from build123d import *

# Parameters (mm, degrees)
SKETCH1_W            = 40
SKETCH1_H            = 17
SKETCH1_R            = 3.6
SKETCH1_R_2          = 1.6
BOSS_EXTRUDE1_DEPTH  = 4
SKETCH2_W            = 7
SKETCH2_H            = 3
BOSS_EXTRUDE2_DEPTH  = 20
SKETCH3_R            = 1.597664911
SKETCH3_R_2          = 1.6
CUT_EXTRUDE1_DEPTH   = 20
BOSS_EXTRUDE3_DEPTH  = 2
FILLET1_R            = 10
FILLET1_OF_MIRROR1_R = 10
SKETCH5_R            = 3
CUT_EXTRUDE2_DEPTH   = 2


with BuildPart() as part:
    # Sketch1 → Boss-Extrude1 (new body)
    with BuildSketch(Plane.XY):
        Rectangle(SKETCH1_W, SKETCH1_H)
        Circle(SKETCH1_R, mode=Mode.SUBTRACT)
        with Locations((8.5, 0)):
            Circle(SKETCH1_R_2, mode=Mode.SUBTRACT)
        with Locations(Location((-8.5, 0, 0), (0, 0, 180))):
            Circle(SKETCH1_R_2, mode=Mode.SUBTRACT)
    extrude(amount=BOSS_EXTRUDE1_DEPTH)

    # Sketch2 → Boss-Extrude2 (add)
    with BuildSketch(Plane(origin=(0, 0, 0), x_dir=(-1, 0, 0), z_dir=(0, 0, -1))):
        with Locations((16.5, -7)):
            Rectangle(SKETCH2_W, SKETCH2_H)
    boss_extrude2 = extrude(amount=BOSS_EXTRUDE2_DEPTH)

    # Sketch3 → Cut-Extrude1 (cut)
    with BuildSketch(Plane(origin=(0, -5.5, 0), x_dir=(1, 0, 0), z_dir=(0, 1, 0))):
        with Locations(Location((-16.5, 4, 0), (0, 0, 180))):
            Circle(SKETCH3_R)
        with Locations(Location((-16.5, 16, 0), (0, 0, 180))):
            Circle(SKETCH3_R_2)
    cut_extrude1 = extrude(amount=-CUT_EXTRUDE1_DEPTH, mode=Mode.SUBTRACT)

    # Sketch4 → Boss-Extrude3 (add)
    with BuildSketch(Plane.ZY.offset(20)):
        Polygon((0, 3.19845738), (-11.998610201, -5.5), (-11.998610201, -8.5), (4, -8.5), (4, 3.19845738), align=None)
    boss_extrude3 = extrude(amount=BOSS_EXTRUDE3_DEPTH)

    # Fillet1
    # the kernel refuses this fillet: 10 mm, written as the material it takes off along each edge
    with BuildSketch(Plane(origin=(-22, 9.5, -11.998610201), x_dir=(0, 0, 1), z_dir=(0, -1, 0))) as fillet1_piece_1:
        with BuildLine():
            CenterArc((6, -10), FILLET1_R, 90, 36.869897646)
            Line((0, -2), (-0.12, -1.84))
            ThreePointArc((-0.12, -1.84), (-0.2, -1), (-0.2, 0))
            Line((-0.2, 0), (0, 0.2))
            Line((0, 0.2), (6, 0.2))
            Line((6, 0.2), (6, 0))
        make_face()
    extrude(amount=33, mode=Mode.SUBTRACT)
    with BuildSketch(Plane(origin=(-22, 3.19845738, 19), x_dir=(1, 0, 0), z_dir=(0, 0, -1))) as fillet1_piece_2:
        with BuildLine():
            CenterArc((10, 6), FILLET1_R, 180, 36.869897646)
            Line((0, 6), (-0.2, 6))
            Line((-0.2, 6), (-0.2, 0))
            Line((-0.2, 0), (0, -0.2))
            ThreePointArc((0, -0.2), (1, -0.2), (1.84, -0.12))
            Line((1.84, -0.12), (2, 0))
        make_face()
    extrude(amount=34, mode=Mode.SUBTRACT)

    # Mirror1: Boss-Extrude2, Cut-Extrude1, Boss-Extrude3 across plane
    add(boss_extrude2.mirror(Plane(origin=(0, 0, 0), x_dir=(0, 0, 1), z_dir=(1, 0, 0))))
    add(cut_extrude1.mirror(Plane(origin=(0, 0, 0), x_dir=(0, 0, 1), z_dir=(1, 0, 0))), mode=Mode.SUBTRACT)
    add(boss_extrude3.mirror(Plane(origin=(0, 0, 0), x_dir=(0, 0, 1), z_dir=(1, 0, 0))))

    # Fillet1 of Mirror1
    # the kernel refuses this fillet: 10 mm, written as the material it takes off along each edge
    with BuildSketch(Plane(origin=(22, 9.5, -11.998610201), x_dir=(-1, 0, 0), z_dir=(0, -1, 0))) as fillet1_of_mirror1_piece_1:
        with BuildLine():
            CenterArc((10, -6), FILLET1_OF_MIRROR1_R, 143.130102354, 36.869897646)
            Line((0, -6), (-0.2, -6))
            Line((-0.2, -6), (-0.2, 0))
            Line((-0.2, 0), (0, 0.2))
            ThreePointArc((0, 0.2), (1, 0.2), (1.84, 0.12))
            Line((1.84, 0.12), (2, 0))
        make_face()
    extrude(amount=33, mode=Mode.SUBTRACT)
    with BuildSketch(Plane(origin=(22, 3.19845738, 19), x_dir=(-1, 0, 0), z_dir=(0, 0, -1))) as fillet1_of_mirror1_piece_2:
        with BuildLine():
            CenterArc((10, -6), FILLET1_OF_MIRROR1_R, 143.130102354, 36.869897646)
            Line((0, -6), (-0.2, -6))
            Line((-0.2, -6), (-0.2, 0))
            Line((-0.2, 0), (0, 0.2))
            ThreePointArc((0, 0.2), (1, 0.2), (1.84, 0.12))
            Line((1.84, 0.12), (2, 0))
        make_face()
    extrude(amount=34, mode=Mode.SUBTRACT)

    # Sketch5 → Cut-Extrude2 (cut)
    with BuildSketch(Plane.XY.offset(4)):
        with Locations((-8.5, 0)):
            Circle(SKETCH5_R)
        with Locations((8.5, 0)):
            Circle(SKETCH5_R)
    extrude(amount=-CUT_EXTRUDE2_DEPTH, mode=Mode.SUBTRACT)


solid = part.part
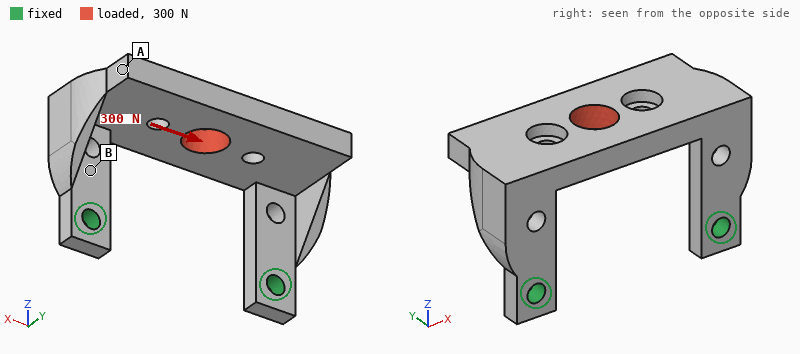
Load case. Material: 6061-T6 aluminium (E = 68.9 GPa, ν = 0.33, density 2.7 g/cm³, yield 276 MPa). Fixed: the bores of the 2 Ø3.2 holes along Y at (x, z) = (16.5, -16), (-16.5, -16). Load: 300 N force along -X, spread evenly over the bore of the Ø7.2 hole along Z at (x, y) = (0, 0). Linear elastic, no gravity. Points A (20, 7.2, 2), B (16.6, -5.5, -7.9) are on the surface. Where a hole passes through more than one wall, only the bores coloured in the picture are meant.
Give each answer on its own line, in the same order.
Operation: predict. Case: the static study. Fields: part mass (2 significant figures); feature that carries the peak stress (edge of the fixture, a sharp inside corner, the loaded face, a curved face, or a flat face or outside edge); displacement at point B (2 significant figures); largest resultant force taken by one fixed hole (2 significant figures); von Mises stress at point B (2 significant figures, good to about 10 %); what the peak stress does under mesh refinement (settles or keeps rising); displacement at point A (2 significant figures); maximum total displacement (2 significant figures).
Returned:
9.8 g
edge of the fixture
14 µm
170 N
31 MPa
keeps rising
52 µm
55 µm
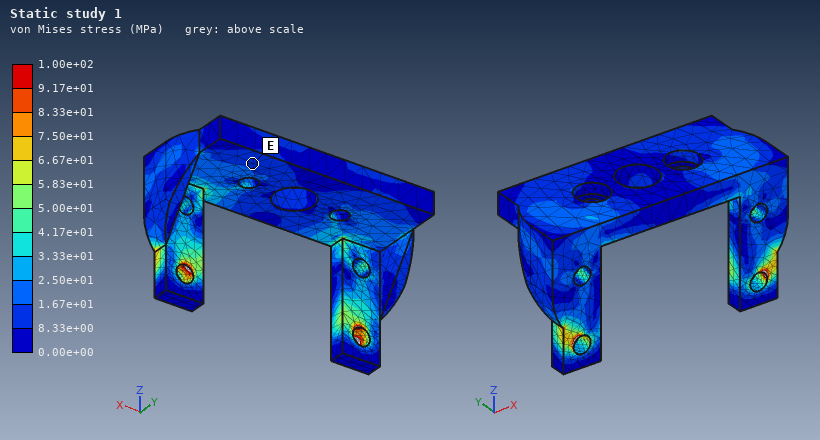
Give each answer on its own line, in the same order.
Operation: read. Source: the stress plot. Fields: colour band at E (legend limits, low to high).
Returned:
8.33e+00 to 1.67e+01 MPa
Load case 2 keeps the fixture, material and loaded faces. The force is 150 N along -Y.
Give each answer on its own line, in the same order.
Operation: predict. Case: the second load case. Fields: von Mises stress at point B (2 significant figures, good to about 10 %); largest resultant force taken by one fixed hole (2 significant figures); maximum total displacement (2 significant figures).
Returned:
38 MPa
75 N
0.16 mm
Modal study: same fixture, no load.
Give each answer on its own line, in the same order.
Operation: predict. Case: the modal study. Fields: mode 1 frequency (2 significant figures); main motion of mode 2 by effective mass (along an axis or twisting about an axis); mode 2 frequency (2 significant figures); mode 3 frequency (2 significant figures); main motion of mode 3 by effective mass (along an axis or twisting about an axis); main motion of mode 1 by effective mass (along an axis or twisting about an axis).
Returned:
1900 Hz
along X
4200 Hz
6100 Hz
along X
along Y
